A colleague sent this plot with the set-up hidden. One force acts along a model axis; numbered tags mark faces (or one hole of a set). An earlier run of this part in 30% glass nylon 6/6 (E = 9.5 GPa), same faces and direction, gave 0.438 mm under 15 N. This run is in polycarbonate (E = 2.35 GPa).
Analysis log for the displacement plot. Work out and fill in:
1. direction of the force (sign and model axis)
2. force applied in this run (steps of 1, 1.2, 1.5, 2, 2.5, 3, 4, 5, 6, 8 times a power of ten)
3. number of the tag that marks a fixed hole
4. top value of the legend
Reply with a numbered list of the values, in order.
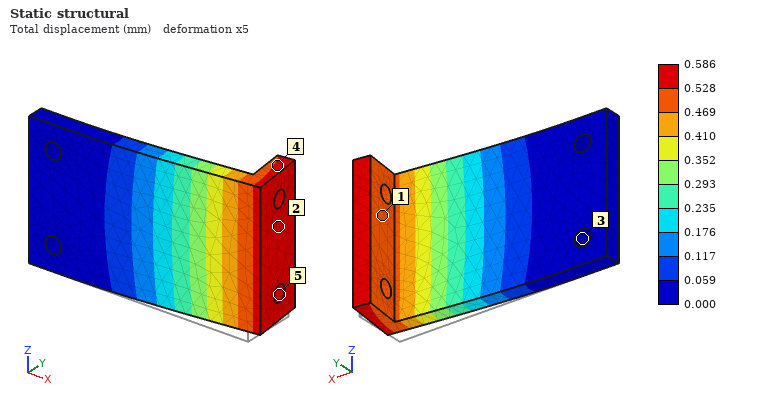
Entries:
1. +Y
2. 5 N
3. 3
4. 0.586 mm
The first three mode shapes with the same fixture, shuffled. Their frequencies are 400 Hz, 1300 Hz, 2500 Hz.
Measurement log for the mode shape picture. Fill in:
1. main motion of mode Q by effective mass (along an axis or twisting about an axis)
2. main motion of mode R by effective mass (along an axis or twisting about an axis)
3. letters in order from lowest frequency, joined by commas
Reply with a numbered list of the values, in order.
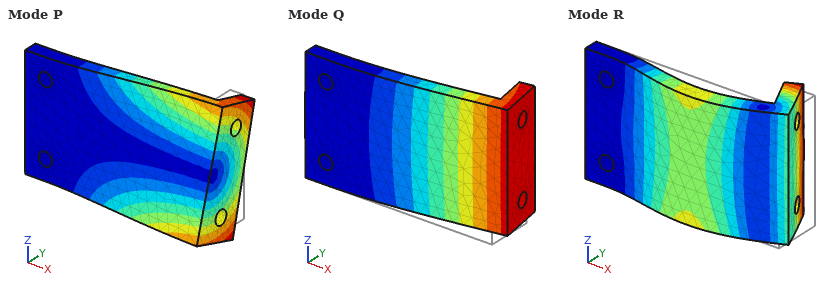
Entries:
1. along Y
2. along Y
3. Q, P, R
